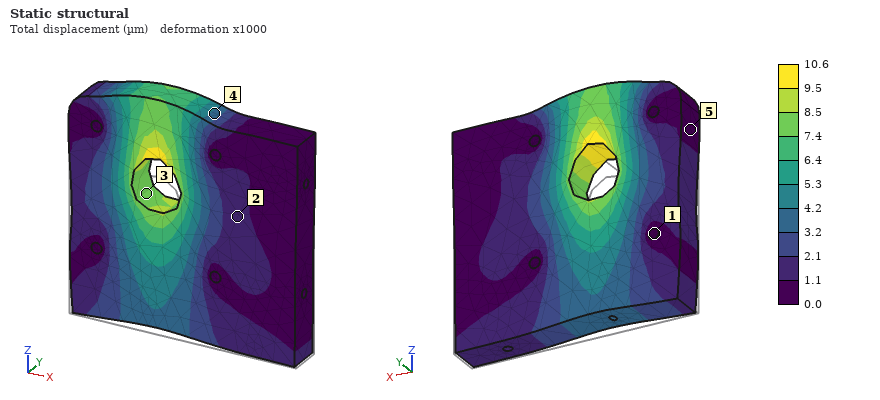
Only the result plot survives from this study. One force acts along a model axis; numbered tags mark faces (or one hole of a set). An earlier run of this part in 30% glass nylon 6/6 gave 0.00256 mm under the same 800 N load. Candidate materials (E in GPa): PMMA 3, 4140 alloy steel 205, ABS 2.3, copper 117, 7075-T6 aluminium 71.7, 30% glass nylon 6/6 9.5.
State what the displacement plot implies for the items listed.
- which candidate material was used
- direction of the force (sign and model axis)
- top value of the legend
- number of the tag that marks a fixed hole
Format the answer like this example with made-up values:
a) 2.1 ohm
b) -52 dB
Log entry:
a) ABS
b) +Z
c) 10.6 µm
d) 1
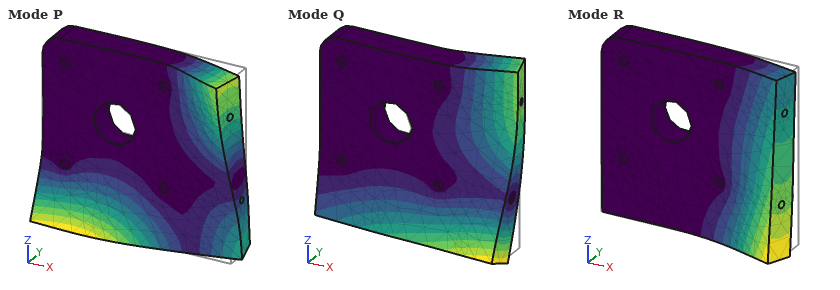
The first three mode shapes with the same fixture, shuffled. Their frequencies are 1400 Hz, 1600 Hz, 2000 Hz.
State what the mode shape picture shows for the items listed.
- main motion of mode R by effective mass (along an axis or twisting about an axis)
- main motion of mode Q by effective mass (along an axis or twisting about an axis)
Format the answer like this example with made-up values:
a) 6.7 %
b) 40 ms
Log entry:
a) along Y
b) twisting about X
